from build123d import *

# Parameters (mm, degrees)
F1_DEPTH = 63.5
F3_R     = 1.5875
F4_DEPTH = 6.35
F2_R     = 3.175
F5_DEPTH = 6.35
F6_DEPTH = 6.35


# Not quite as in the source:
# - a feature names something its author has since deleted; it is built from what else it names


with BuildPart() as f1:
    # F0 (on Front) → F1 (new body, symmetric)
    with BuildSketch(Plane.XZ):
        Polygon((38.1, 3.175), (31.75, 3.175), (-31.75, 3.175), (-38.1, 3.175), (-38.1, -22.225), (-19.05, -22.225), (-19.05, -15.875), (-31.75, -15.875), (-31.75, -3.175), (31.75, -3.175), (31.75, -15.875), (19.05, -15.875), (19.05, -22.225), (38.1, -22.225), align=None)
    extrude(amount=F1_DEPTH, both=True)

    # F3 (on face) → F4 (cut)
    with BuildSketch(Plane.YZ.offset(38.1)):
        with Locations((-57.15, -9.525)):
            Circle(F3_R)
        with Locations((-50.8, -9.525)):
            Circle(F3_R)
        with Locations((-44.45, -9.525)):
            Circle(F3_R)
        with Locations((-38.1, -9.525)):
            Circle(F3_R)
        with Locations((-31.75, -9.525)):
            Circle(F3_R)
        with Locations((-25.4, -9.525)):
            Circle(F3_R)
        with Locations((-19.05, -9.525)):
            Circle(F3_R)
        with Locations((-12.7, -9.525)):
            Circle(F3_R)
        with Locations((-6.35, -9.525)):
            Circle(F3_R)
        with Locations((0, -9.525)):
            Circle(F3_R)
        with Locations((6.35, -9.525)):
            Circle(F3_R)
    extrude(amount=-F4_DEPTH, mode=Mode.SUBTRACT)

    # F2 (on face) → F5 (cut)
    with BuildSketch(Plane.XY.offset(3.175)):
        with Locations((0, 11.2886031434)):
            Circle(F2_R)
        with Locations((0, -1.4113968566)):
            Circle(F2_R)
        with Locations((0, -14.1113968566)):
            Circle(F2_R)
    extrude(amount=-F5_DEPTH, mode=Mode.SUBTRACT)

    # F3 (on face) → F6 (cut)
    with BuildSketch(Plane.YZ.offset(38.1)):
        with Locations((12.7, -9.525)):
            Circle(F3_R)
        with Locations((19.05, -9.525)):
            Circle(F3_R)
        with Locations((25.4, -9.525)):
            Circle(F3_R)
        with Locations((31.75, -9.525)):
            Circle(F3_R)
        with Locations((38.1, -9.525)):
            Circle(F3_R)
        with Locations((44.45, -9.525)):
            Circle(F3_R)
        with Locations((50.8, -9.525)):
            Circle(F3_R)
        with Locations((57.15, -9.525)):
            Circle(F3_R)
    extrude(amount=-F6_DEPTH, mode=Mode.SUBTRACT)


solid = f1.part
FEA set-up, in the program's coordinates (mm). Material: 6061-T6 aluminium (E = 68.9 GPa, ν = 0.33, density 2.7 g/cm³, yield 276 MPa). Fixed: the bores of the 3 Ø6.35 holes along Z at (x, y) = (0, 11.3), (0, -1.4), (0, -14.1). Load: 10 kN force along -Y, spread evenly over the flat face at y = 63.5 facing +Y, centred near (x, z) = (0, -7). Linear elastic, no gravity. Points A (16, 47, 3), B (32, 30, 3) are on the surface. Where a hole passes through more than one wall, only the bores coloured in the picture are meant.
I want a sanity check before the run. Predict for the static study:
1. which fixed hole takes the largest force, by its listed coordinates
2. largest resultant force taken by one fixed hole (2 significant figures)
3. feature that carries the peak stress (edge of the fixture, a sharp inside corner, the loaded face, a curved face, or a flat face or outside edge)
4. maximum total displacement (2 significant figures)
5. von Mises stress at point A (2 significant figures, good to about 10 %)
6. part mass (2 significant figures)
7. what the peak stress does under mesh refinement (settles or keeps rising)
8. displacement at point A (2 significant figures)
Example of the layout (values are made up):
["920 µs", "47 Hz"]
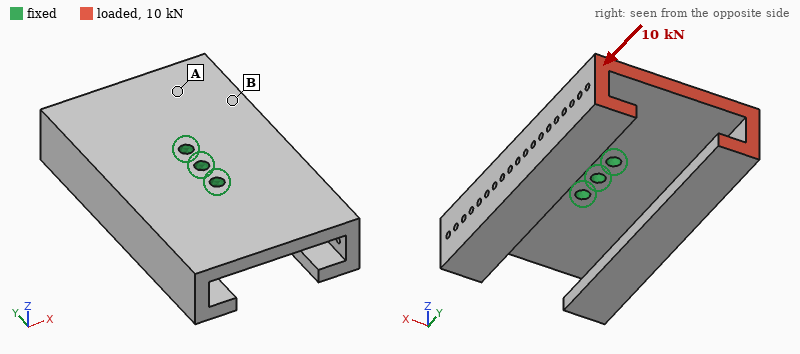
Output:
["(0, 11.3)", "5.1 kN", "edge of the fixture", "0.22 mm", "23 MPa", "300 g", "keeps rising", "0.11 mm"]
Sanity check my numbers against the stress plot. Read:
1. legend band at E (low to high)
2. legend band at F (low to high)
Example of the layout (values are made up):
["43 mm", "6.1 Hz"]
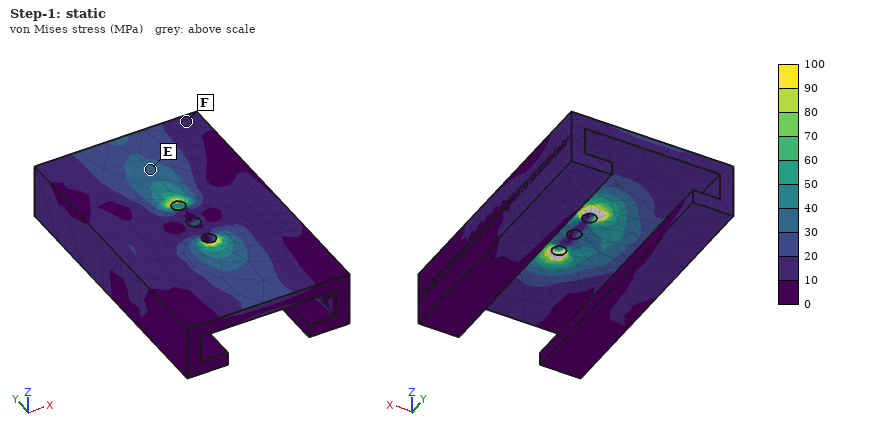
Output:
["30 to 40 MPa", "10 to 20 MPa"]
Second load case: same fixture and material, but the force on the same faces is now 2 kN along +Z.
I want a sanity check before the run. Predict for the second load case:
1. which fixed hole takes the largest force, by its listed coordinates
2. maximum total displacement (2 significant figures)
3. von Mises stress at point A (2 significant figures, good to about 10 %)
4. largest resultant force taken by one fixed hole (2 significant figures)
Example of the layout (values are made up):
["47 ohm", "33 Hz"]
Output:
["(0, 11.3)", "0.43 mm", "29 MPa", "4.2 kN"]
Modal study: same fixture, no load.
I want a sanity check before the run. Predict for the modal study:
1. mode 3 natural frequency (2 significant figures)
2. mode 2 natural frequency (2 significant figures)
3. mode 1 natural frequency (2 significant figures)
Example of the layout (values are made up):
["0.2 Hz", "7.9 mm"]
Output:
["1500 Hz", "1300 Hz", "1300 Hz"]
